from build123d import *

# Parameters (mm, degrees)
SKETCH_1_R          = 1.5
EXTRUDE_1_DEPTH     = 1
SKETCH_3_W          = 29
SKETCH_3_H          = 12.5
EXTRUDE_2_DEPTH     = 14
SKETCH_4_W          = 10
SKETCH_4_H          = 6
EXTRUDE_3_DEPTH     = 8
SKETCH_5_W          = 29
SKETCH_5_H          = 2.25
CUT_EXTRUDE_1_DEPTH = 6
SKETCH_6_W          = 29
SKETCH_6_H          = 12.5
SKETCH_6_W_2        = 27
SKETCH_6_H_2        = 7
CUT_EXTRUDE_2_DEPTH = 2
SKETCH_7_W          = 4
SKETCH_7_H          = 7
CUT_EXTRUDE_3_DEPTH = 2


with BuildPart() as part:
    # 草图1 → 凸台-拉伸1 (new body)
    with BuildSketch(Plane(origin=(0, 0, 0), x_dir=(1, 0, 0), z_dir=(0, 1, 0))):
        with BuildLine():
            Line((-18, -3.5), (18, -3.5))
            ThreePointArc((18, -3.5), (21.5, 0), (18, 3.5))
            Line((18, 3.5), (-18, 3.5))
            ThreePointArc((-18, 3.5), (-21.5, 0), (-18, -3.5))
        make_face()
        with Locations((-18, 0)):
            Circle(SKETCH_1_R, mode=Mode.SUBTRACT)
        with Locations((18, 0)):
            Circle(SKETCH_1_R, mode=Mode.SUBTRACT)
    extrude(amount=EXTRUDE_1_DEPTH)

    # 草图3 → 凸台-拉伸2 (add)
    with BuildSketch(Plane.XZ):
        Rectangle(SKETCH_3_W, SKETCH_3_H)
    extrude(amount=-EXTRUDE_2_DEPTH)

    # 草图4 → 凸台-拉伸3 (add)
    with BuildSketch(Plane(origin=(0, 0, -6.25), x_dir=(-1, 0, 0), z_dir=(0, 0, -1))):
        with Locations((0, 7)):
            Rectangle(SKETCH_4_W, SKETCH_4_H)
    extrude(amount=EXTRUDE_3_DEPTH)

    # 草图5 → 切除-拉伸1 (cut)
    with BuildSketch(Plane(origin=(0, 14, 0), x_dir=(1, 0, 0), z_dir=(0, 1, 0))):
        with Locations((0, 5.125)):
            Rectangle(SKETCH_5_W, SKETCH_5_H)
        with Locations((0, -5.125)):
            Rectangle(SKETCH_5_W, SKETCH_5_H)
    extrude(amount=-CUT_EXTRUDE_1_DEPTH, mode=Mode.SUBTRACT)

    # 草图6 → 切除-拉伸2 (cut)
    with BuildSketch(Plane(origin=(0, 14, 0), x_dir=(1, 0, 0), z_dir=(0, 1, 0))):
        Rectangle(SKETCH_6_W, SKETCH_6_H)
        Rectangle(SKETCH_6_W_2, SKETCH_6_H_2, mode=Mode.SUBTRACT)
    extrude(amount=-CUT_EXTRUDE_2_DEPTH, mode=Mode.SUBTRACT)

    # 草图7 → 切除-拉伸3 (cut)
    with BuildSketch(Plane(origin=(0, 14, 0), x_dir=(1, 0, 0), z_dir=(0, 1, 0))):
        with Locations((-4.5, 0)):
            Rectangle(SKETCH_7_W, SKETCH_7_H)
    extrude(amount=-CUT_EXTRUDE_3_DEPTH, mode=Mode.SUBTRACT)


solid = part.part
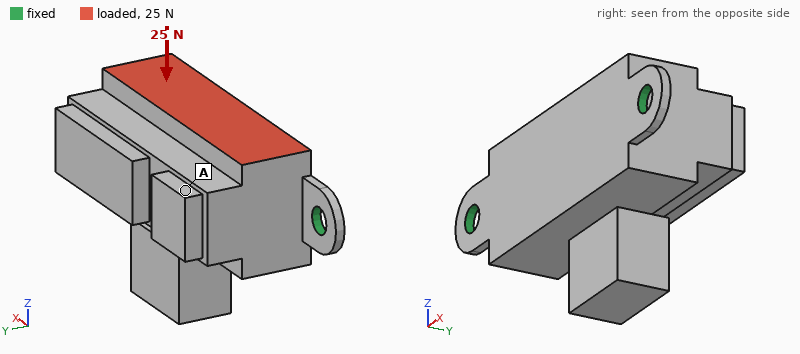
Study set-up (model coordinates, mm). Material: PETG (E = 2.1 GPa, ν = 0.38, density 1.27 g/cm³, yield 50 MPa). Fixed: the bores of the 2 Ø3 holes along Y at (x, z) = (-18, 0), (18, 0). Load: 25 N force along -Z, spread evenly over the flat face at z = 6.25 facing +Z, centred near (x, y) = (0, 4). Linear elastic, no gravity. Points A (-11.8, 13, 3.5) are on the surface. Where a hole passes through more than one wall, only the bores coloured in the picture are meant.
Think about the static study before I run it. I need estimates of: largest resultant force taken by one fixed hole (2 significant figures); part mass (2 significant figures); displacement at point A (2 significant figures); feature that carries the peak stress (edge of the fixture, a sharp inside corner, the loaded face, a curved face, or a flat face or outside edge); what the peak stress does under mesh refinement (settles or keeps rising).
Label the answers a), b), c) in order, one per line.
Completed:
a) 13 N
b) 6.0 g
c) 0.42 mm
d) edge of the fixture
e) keeps rising
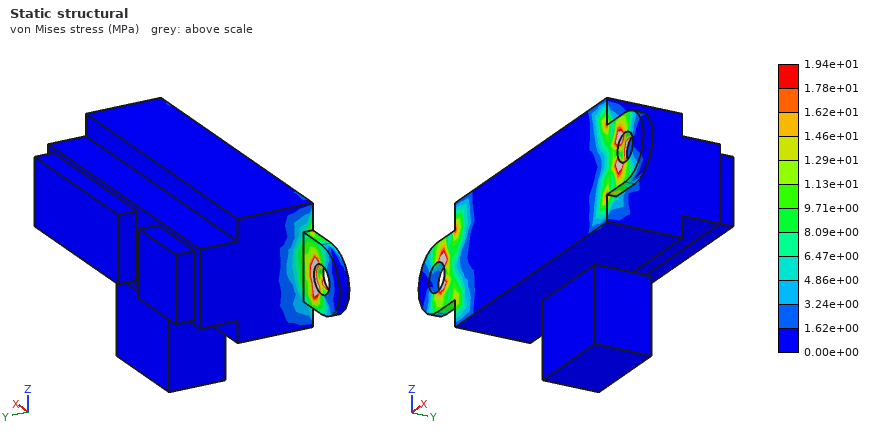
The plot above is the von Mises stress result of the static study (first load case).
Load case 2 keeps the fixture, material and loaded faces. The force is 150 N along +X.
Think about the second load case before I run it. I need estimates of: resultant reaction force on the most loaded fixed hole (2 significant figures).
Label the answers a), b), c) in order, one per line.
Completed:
a) 82 N
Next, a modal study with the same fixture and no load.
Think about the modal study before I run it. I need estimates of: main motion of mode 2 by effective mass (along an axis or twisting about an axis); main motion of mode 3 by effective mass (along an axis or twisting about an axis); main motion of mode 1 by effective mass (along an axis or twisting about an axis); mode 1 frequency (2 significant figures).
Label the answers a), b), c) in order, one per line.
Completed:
a) along Y
b) along X
c) along Z
d) 430 Hz
